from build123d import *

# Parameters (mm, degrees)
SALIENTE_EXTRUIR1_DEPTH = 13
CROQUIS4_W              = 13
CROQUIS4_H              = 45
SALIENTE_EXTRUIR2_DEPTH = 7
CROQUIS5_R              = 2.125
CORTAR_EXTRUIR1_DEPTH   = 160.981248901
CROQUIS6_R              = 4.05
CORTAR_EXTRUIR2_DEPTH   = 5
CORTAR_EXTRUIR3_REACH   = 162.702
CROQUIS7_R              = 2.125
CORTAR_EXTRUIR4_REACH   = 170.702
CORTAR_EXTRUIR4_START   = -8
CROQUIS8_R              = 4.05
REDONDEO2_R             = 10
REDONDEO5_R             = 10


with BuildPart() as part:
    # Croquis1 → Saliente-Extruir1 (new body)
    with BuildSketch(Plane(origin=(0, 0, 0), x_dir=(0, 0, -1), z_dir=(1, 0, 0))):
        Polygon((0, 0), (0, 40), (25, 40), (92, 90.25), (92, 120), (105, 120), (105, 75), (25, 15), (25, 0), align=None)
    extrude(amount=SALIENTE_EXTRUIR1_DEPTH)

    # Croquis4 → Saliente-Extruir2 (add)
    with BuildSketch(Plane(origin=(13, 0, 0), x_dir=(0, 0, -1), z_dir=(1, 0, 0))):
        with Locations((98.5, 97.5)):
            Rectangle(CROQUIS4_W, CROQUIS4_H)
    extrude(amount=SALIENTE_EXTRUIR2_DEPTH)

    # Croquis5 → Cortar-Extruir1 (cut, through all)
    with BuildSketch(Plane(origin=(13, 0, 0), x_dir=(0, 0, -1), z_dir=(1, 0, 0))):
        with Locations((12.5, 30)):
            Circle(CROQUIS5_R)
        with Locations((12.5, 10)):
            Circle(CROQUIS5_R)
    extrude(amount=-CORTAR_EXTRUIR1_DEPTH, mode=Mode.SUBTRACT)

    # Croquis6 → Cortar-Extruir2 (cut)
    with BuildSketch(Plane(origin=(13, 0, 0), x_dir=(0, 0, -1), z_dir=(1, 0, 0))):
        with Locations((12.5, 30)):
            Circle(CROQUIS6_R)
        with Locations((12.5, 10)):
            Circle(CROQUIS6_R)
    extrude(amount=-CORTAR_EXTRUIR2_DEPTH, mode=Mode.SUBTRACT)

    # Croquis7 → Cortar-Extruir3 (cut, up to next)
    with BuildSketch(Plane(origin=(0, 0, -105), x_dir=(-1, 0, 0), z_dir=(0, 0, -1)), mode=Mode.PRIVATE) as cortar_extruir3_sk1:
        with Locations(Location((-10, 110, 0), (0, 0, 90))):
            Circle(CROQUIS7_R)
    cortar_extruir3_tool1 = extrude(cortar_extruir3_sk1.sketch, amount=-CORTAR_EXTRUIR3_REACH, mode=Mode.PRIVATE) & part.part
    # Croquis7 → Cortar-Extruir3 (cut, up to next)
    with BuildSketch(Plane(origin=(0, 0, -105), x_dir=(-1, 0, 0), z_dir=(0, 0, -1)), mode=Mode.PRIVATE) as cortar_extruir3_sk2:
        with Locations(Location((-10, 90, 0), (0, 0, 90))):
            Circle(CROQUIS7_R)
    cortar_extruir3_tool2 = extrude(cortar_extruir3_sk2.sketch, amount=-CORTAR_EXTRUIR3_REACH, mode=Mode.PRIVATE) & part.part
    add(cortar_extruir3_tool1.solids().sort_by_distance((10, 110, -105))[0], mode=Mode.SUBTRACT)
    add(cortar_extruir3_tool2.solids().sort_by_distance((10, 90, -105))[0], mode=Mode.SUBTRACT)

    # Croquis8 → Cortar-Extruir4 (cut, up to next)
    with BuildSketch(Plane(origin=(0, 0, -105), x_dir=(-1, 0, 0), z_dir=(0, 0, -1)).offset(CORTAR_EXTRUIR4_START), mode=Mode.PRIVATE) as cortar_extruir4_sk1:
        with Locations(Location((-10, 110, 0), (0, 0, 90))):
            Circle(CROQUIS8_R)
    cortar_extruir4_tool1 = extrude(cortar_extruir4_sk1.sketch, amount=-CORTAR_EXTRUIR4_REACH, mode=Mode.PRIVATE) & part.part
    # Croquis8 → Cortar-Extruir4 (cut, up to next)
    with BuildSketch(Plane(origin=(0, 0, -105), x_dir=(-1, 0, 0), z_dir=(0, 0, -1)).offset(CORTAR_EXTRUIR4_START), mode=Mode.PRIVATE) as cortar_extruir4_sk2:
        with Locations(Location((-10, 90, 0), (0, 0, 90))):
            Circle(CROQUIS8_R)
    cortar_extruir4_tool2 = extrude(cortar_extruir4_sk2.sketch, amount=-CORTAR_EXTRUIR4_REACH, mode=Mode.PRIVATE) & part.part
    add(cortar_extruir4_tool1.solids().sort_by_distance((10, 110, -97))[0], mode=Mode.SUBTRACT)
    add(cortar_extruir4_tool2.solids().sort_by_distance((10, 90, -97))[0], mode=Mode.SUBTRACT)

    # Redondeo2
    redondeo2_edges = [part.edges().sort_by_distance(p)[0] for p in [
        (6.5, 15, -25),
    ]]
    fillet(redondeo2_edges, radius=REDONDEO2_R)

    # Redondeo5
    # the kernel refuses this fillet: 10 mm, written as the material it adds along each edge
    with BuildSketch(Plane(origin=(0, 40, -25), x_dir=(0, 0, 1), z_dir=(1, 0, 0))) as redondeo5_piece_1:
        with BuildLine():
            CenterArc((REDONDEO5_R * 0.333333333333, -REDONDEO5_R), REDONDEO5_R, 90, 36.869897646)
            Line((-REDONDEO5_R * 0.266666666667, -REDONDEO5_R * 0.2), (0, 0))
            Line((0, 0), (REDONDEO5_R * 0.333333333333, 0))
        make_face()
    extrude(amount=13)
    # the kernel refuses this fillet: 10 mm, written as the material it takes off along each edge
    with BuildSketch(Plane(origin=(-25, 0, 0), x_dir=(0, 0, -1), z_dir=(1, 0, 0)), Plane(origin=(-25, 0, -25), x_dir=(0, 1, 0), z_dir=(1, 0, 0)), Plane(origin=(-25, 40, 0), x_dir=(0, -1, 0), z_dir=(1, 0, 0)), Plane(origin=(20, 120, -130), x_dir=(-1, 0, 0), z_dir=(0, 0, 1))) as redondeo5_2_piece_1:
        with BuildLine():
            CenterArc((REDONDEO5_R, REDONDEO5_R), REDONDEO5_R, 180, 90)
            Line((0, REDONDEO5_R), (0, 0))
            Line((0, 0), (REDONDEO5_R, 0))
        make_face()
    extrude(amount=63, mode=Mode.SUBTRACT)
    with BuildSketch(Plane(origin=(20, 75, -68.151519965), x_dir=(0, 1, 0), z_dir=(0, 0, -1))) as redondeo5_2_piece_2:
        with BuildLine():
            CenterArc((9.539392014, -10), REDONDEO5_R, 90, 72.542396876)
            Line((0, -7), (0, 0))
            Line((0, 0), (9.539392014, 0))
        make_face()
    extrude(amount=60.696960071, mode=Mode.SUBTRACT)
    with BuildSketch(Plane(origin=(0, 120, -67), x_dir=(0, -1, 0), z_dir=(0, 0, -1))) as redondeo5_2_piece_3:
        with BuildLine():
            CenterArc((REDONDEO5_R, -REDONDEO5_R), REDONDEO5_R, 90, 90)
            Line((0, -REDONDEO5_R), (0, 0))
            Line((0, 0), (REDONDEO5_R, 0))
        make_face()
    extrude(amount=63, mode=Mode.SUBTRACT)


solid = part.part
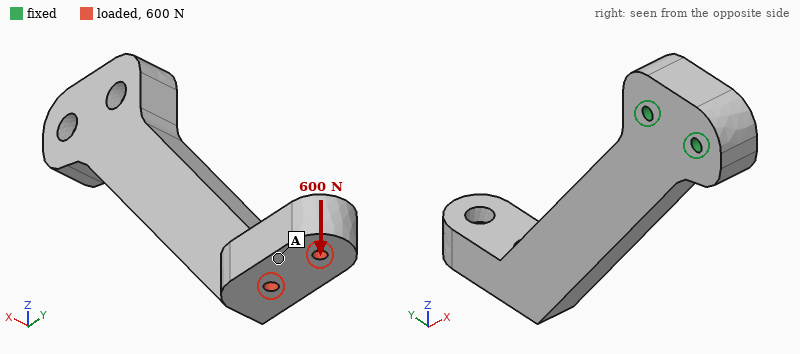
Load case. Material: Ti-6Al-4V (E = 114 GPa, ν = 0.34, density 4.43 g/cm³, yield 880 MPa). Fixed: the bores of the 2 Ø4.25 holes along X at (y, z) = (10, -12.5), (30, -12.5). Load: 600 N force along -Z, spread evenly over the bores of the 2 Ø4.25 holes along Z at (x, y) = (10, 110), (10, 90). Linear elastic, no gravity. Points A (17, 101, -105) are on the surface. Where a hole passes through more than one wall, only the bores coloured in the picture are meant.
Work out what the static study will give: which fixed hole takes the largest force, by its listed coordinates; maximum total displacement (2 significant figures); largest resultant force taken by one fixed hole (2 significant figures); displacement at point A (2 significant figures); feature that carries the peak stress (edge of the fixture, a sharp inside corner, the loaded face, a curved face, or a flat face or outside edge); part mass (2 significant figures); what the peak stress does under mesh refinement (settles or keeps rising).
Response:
(30, -12.5)
0.27 mm
2.5 kN
0.23 mm
edge of the fixture
200 g
keeps rising
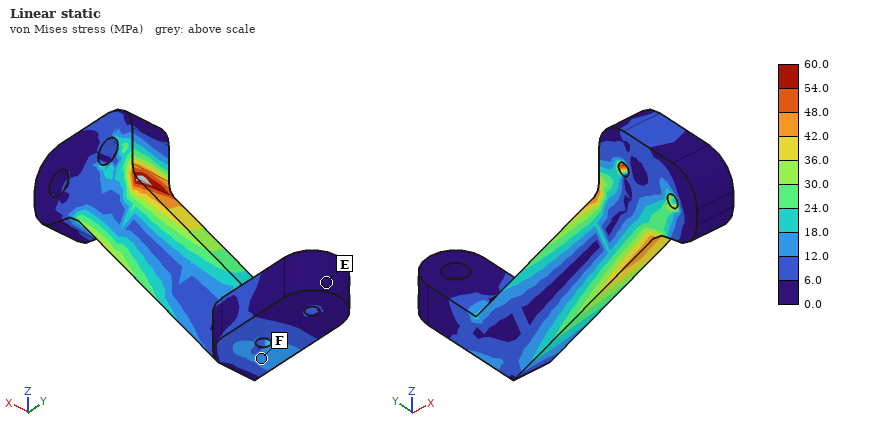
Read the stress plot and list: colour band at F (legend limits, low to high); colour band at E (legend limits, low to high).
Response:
12.0 to 18.0 MPa
0.0 to 6.0 MPa
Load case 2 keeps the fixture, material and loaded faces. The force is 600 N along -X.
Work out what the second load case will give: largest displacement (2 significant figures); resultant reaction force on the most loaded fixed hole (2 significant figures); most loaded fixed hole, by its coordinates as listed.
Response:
0.97 mm
2.2 kN
(30, -12.5)
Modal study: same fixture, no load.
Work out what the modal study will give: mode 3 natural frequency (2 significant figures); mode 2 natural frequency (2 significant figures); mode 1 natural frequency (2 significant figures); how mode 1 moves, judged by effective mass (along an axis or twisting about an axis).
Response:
2700 Hz
970 Hz
570 Hz
along X
